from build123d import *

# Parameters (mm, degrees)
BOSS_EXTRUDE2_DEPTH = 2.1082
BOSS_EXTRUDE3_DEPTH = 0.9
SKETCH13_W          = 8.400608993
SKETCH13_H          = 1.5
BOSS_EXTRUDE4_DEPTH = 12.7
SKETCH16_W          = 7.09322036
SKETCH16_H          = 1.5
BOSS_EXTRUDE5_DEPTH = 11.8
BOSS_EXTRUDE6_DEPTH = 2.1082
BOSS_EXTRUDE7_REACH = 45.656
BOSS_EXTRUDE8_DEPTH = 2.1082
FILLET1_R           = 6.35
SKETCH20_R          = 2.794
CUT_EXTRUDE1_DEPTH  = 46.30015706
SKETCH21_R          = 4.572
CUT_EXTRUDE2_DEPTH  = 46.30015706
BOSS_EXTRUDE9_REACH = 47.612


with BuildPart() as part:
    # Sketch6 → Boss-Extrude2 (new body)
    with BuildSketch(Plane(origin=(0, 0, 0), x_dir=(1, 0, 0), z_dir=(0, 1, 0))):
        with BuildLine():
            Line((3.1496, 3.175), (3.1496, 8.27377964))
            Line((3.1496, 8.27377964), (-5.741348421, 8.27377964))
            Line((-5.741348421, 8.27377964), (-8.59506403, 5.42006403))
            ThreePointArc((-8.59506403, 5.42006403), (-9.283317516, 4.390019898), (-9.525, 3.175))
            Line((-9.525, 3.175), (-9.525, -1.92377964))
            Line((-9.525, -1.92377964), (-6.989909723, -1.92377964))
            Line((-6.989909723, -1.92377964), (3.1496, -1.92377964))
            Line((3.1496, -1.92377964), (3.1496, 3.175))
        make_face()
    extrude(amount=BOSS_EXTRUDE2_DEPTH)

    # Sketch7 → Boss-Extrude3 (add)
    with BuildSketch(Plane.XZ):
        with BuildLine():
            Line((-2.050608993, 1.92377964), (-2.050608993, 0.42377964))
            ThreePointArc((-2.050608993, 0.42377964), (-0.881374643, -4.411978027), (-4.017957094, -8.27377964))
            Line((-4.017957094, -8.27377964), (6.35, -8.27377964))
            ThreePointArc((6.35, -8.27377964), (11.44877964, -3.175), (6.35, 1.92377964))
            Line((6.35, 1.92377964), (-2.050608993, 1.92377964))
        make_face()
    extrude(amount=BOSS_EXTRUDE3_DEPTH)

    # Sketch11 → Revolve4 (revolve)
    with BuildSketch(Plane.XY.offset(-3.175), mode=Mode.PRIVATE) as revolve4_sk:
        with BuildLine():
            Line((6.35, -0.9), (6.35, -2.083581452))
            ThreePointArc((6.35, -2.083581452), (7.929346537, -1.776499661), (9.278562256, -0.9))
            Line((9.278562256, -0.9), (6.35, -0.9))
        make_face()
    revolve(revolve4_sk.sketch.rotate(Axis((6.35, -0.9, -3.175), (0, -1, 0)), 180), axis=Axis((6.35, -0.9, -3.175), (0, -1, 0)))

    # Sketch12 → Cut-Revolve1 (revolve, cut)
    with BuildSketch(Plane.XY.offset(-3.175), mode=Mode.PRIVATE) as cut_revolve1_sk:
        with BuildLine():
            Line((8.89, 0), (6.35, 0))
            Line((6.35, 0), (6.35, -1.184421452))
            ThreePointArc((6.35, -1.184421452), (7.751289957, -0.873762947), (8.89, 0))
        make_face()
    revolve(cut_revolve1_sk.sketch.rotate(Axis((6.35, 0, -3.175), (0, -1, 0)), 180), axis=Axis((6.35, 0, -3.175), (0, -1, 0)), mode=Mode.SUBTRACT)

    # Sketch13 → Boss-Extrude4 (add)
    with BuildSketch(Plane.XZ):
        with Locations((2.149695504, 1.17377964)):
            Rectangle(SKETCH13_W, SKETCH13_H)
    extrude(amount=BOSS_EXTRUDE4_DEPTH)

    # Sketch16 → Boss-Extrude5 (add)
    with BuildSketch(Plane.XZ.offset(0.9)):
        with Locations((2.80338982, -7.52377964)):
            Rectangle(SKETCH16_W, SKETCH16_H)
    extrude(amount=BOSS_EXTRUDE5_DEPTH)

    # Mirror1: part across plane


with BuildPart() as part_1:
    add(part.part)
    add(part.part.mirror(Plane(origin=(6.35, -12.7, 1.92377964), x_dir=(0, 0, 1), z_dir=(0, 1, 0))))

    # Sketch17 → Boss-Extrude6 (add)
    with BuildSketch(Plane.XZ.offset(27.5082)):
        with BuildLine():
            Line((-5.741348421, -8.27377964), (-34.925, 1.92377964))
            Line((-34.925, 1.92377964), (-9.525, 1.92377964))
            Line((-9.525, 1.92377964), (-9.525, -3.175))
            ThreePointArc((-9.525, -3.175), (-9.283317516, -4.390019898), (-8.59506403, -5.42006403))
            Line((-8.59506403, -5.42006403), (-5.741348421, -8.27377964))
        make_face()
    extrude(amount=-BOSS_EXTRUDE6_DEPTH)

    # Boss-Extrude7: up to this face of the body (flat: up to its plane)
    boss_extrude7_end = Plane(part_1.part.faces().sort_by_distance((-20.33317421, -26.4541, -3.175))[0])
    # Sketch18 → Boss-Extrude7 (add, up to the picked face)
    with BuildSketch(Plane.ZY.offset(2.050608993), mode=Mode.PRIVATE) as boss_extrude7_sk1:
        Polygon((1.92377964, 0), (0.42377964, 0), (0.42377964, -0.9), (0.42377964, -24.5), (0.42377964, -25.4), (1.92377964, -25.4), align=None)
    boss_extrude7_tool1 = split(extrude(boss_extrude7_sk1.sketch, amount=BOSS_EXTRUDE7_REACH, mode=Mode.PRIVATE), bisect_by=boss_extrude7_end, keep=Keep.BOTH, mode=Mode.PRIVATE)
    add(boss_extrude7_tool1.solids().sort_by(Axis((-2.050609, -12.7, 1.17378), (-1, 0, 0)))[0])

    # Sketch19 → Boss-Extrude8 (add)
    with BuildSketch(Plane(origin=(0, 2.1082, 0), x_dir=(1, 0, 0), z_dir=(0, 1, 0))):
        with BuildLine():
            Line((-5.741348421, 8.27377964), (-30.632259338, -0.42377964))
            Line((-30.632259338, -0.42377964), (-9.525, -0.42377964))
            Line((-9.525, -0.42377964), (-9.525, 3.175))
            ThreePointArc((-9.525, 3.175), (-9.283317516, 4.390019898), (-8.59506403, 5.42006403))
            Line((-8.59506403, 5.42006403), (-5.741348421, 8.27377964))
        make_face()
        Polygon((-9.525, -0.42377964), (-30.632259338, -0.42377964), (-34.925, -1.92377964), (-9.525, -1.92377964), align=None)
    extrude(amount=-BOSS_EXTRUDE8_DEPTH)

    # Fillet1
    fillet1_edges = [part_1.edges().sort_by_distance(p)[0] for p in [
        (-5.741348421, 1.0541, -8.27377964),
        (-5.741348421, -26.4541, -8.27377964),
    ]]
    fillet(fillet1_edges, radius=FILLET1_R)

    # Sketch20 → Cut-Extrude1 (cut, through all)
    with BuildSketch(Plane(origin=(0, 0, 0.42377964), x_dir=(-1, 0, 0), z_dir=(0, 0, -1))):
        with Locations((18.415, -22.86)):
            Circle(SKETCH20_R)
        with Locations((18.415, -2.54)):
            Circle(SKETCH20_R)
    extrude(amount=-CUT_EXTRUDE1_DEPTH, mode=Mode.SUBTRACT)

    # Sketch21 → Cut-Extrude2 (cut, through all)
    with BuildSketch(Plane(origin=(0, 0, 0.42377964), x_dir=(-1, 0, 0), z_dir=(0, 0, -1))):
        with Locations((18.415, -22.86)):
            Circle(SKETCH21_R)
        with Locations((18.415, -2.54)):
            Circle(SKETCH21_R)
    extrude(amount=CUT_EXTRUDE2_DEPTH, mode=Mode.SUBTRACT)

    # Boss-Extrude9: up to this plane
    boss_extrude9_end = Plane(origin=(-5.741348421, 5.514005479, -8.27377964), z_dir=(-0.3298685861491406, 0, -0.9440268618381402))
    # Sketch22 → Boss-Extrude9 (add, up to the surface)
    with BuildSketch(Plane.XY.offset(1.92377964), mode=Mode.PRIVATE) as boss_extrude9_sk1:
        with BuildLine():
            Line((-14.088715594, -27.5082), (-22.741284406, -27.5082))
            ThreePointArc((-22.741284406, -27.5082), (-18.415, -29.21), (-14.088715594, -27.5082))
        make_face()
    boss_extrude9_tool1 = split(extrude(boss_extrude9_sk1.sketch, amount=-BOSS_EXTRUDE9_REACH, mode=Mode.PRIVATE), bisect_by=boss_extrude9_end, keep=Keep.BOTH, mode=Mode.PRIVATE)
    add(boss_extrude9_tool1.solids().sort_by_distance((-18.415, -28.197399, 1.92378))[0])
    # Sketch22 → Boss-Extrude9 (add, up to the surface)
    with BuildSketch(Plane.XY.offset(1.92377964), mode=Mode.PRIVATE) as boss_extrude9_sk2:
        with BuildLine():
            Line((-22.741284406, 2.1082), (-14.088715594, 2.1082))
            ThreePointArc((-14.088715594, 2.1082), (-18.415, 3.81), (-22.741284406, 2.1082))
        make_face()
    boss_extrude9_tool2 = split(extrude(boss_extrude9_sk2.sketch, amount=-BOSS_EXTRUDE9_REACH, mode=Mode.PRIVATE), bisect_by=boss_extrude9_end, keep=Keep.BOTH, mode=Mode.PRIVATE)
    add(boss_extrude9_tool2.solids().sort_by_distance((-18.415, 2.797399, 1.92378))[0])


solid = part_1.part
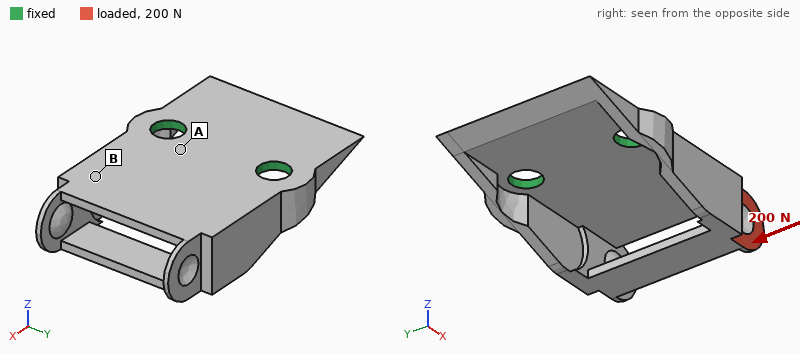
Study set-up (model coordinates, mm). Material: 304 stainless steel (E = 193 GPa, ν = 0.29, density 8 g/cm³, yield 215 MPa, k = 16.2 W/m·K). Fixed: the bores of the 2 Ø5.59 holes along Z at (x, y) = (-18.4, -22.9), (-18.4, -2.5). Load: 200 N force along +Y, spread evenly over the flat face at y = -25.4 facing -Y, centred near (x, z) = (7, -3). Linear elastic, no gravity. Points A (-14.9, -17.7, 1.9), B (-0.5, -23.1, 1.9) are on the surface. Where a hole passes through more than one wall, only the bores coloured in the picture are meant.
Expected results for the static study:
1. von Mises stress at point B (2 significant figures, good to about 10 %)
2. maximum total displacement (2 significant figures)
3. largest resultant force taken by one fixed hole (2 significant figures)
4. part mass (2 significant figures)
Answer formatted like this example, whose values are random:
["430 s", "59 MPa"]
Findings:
["23 MPa", "44 µm", "240 N", "23 g"]
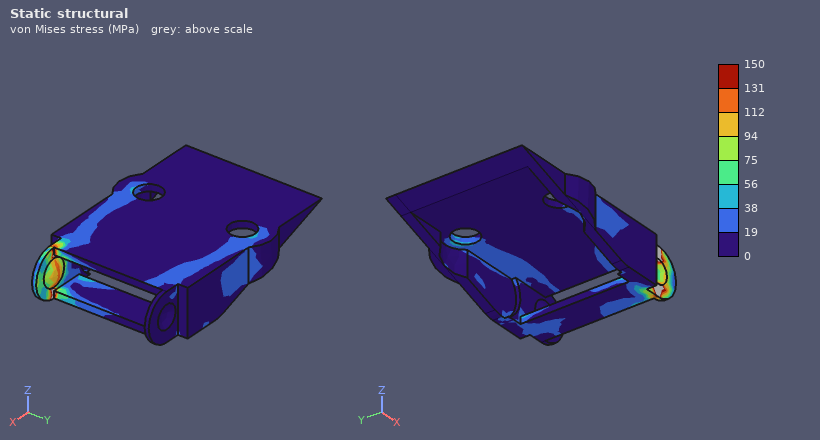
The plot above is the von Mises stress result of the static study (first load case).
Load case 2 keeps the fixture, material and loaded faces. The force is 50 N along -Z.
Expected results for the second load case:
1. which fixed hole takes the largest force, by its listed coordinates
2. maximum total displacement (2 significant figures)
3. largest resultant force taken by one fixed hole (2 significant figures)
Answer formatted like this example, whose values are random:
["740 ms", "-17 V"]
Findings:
["(-18.4, -22.9)", "39 µm", "51 N"]
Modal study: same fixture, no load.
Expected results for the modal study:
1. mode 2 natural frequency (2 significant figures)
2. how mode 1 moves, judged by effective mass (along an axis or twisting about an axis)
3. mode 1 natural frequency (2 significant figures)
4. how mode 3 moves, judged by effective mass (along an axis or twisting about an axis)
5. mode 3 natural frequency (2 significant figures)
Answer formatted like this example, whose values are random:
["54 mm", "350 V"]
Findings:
["4300 Hz", "along Z", "3100 Hz", "along Y", "7900 Hz"]
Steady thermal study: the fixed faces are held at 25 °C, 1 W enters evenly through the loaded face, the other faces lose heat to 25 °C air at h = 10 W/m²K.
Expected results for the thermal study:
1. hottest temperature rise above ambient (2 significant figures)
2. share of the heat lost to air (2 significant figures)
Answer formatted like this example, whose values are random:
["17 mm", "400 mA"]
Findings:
["45 K", "30 %"]
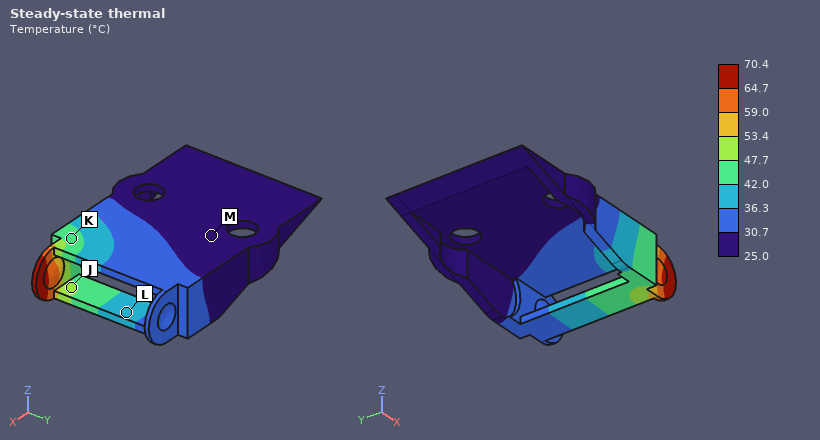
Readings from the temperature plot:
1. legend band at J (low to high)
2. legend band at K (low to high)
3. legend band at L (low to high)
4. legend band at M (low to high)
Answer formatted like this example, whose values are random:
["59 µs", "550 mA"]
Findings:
["47.7 to 53.4 °C", "42.0 to 47.7 °C", "36.3 to 42.0 °C", "25.0 to 30.7 °C"]
